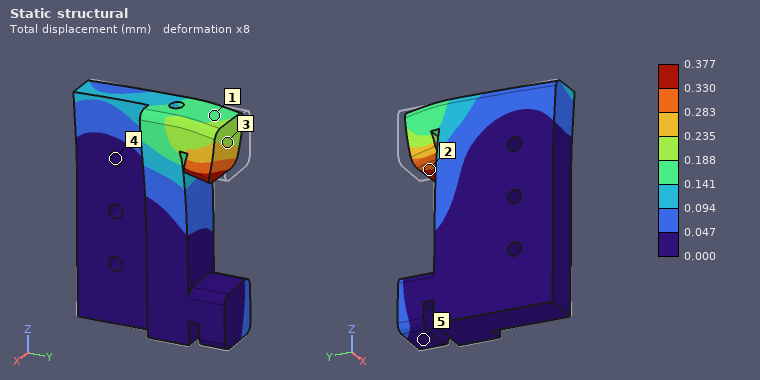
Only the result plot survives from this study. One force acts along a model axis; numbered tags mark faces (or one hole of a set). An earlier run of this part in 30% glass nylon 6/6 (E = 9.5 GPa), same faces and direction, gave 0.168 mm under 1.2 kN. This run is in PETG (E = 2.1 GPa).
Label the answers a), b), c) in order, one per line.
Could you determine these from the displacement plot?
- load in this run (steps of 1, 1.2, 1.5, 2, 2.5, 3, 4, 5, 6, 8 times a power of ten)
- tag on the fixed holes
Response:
a) 600 N
b) 4
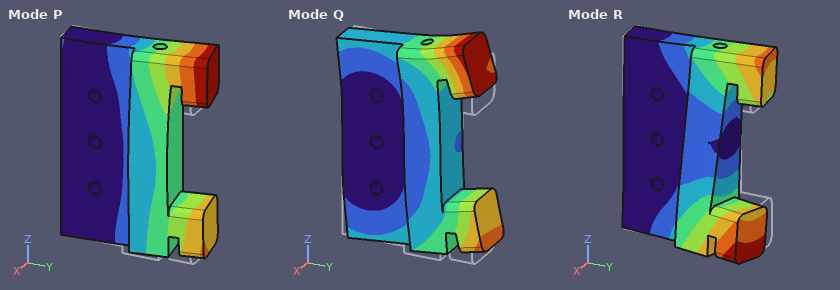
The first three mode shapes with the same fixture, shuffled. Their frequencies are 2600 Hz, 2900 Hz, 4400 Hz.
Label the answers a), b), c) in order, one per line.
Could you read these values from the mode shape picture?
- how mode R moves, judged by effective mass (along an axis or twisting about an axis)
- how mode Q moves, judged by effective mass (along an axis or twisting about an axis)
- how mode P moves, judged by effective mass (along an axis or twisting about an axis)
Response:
a) twisting about Y
b) along Z
c) along X
